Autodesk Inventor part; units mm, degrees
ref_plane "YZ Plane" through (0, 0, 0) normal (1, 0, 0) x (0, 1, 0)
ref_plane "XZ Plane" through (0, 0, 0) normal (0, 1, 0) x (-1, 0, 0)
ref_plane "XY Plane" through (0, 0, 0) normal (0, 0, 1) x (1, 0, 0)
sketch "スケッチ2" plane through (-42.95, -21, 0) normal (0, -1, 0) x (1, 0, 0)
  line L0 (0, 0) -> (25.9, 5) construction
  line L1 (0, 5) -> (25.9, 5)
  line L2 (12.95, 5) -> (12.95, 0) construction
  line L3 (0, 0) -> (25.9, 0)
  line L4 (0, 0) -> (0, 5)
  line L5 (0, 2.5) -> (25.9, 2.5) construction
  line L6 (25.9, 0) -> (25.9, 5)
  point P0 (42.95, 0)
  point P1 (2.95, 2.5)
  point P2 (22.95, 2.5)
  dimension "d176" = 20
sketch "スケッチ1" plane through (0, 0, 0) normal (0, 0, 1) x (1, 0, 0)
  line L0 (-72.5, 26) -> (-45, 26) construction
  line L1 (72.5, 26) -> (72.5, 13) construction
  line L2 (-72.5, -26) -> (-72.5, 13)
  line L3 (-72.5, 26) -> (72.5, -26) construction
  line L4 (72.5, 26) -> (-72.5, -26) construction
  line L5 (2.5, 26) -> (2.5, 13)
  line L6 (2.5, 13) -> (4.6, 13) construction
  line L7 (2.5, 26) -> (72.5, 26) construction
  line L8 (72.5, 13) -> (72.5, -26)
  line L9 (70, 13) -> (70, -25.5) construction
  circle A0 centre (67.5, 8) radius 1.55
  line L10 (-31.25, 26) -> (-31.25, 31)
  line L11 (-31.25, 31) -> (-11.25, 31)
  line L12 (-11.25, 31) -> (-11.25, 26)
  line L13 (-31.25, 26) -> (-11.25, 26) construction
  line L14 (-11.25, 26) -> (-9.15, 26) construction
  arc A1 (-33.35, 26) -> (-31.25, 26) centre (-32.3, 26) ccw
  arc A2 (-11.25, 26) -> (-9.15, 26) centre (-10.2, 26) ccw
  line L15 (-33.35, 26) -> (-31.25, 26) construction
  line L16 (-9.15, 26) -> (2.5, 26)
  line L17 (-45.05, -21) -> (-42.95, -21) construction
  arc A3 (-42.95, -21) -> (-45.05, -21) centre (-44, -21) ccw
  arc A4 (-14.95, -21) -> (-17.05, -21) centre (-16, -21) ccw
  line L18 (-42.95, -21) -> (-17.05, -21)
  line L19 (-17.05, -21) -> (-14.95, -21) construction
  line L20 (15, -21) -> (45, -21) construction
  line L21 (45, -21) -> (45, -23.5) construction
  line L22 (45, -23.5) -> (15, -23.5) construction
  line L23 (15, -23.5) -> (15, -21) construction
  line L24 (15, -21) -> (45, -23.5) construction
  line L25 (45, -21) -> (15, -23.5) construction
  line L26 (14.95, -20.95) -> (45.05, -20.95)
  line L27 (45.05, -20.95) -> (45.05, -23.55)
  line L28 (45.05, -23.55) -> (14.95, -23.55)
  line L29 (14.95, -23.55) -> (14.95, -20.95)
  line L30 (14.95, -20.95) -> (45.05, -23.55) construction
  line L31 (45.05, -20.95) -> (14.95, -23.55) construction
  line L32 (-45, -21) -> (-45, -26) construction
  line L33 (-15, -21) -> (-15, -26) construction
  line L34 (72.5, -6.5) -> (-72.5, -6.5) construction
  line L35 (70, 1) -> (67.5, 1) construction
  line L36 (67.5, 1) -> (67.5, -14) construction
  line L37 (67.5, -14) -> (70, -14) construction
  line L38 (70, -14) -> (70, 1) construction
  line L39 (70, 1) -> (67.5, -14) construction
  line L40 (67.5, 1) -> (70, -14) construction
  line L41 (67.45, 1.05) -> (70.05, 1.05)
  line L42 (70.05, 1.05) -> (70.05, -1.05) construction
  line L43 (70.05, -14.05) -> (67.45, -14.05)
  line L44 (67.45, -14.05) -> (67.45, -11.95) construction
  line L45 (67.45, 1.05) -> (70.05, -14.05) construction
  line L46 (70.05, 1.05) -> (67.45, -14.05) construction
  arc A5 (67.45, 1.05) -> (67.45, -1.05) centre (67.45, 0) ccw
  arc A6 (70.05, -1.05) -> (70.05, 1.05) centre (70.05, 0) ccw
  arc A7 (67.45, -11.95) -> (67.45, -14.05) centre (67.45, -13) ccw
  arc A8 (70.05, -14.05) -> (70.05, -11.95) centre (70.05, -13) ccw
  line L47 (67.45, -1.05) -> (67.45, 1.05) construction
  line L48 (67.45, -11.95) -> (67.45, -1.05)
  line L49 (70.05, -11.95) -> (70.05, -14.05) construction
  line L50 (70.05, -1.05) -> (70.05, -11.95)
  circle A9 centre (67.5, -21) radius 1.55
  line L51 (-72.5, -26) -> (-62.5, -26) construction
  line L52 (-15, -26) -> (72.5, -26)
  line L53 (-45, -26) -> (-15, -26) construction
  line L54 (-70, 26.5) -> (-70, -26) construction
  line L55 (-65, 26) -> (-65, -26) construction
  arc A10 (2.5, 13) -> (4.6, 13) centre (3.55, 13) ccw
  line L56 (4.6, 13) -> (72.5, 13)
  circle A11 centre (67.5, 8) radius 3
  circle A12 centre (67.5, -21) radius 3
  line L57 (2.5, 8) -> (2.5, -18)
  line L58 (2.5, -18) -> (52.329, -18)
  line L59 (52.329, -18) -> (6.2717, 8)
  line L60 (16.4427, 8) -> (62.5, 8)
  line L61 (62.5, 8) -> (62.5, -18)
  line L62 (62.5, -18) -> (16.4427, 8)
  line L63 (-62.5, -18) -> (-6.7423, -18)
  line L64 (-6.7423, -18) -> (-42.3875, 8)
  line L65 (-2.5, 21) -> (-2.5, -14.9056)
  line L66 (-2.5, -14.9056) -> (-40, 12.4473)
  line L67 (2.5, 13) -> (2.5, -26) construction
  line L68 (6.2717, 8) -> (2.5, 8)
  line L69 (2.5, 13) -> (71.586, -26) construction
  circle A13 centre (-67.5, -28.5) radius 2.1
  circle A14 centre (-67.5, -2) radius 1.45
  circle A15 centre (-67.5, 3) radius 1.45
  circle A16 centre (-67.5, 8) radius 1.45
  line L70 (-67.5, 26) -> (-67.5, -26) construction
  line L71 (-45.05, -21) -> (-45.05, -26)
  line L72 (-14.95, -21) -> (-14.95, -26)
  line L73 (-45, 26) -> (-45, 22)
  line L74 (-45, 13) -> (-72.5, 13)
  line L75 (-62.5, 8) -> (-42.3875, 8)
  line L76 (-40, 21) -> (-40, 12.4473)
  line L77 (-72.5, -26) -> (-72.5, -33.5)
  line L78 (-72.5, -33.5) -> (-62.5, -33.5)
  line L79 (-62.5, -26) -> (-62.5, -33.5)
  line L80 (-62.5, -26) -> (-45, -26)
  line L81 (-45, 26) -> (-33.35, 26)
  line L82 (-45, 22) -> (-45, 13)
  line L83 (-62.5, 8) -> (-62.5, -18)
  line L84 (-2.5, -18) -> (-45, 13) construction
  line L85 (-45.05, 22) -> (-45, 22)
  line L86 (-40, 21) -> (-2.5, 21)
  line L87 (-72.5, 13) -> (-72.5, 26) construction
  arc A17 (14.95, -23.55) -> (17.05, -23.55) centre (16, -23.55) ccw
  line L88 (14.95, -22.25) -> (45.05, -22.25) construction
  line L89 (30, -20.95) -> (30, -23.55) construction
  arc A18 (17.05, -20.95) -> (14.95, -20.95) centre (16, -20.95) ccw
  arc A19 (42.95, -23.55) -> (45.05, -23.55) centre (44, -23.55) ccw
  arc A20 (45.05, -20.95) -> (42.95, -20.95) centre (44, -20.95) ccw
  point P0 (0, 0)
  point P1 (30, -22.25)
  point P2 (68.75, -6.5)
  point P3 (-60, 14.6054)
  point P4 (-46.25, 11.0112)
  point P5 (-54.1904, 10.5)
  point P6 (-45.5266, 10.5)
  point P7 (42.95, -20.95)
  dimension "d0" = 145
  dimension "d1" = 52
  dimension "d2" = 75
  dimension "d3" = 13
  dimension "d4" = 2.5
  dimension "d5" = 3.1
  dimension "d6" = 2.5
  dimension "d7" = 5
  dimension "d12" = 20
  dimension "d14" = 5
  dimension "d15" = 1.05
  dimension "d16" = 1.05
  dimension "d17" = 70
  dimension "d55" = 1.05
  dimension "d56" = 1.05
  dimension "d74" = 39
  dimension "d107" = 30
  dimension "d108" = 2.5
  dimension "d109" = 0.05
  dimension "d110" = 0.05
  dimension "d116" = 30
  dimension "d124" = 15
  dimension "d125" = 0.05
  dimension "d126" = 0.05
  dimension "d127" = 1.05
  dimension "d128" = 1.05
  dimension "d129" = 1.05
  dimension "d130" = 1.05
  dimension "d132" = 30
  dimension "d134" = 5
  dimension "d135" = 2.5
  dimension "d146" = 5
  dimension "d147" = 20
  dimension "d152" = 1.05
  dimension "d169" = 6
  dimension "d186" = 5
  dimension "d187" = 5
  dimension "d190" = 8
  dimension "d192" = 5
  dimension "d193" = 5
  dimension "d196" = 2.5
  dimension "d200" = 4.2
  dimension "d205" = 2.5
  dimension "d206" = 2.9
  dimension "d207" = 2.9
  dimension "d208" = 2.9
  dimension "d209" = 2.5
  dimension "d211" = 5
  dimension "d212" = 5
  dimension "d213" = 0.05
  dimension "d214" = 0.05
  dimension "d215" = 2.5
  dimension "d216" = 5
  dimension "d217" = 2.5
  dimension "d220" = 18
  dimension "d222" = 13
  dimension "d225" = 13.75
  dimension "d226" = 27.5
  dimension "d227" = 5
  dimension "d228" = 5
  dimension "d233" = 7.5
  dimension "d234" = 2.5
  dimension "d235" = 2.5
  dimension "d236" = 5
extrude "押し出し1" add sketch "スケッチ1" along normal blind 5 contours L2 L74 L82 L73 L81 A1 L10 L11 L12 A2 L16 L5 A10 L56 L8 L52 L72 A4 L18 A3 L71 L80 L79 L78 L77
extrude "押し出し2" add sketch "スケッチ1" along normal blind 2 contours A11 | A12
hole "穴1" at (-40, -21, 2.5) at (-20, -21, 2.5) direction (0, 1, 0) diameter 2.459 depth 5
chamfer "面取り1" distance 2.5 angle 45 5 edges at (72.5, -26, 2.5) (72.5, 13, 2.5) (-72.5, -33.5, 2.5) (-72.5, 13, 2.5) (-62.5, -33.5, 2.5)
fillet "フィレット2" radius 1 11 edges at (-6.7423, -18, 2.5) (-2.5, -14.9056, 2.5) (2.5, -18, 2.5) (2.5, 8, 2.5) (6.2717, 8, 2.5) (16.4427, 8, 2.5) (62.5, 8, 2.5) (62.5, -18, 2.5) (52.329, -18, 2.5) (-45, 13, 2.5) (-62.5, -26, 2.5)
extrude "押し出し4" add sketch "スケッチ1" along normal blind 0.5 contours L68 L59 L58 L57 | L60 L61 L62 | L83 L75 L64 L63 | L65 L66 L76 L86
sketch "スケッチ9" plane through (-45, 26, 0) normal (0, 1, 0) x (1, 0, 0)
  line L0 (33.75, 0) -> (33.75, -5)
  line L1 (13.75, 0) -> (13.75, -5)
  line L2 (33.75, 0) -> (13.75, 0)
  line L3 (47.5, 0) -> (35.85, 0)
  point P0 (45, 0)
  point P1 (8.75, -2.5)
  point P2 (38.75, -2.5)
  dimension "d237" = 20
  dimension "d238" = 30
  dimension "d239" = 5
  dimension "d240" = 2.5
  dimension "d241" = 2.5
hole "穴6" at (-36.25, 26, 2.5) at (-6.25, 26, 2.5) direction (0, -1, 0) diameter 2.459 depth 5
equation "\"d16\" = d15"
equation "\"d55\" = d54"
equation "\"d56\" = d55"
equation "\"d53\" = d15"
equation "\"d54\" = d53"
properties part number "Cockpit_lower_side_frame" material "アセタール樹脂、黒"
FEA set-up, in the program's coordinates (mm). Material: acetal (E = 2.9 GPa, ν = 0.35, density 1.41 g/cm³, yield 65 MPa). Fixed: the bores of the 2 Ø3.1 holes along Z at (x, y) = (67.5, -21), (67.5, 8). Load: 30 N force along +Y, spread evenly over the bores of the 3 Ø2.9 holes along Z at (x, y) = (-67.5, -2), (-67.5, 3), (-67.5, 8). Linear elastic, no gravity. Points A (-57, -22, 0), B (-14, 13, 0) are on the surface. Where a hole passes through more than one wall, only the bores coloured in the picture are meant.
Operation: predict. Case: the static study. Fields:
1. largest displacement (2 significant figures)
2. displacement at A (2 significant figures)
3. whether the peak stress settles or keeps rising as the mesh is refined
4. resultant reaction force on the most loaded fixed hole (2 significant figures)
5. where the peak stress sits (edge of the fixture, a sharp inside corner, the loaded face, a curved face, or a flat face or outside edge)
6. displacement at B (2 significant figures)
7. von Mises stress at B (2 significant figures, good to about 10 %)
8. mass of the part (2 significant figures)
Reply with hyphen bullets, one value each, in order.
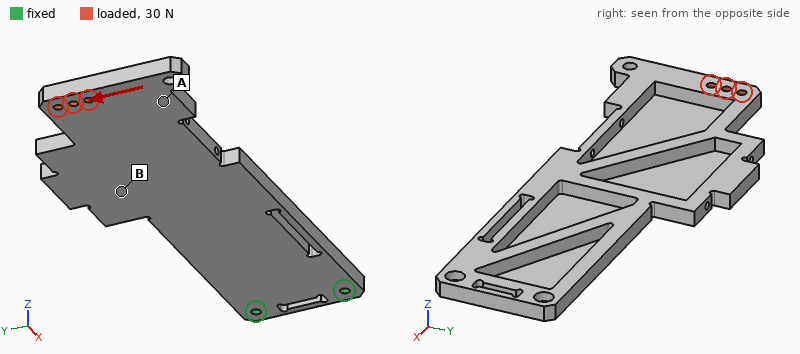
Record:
- 1.7 mm
- 1.2 mm
- keeps rising
- 130 N
- edge of the fixture
- 0.42 mm
- 4.1 MPa
- 23 g
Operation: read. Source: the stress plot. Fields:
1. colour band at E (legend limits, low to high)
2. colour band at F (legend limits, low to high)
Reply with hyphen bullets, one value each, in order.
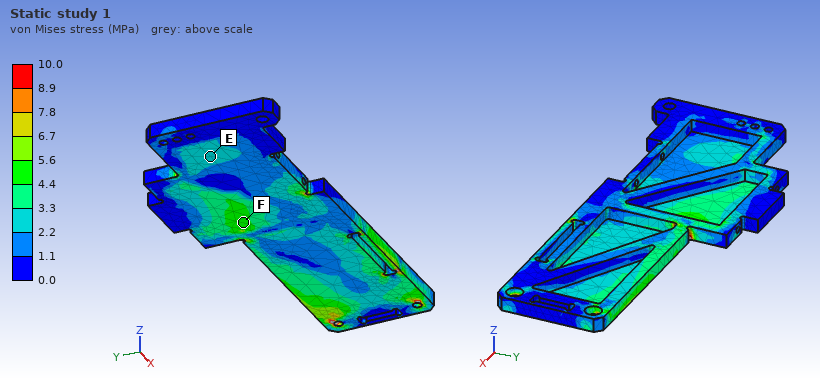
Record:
- 2.2 to 3.3 MPa
- 4.4 to 5.6 MPa
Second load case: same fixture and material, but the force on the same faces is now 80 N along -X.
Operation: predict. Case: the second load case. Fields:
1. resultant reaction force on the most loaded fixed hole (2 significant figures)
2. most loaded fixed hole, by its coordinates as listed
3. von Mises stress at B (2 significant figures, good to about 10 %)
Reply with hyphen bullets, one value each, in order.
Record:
- 64 N
- (67.5, 8)
- 3.4 MPa
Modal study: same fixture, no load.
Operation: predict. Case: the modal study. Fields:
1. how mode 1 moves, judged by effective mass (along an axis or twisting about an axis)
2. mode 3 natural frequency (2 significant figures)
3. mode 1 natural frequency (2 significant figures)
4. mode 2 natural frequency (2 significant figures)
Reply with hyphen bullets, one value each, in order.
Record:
- along Z
- 290 Hz
- 45 Hz
- 170 Hz
